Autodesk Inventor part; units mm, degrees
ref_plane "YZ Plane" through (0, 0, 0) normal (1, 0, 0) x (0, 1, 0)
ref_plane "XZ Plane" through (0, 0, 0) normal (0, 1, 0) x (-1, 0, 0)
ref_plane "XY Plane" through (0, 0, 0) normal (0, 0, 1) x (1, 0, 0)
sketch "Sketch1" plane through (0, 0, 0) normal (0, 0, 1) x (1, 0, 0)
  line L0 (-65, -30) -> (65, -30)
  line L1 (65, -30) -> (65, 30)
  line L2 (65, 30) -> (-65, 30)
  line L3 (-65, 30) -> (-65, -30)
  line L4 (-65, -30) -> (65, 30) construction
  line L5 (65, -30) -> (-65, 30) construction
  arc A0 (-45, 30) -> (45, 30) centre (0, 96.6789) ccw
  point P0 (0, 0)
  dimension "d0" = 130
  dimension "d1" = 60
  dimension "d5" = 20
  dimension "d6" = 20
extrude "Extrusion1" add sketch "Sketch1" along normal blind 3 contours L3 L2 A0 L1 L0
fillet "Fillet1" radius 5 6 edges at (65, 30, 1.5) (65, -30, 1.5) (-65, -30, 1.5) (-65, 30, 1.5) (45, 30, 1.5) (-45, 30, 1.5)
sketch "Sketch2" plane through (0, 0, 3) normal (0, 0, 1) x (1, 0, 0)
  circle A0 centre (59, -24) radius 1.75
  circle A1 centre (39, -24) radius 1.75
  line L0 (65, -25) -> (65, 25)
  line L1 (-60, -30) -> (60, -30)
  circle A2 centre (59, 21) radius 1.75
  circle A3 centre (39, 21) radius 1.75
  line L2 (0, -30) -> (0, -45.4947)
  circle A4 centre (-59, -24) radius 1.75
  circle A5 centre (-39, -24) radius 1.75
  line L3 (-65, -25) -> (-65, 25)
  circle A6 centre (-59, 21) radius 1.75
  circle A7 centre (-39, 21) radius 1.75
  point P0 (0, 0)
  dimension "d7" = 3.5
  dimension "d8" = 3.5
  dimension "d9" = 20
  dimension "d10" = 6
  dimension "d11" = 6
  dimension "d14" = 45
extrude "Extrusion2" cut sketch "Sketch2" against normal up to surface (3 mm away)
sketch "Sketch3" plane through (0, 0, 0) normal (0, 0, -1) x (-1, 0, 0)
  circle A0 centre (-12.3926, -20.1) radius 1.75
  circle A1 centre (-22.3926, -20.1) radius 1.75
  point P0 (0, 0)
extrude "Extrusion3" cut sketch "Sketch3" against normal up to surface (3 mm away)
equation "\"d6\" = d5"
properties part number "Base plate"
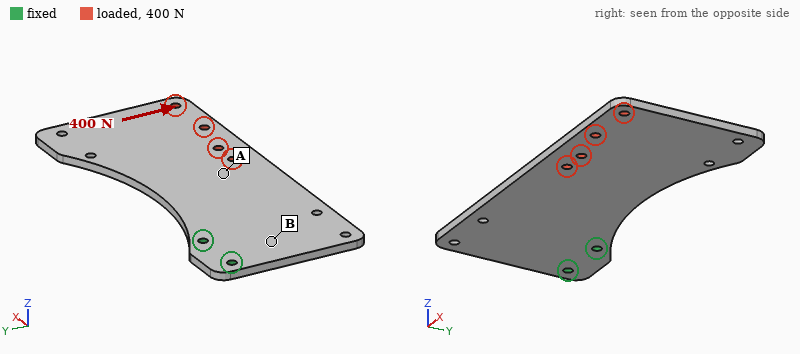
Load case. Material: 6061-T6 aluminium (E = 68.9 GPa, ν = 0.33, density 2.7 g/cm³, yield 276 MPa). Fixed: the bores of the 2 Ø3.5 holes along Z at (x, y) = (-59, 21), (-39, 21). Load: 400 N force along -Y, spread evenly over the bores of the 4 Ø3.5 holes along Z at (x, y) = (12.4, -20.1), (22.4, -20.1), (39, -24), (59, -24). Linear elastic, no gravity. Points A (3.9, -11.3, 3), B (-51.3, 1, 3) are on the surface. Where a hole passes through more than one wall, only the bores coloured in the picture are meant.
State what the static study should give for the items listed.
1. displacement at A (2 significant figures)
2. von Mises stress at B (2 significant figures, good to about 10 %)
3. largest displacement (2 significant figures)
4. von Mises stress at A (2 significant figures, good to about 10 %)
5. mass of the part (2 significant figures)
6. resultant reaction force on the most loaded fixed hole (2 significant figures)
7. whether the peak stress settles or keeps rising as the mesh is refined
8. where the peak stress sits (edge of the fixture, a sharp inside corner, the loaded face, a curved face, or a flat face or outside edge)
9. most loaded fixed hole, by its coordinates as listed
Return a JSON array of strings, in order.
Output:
["0.075 mm", "20 MPa", "0.18 mm", "7.6 MPa", "55 g", "1.7 kN", "keeps rising", "edge of the fixture", "(-39, 21)"]
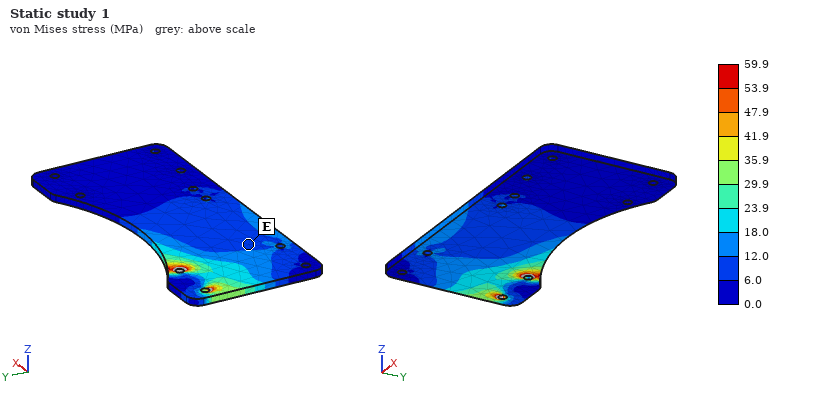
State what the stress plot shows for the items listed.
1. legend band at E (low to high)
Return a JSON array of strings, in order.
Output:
["6.0 to 12.0 MPa"]
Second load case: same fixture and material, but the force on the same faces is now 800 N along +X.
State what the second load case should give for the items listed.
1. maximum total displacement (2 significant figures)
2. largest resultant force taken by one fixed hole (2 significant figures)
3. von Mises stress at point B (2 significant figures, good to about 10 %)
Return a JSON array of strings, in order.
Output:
["0.17 mm", "1.7 kN", "23 MPa"]
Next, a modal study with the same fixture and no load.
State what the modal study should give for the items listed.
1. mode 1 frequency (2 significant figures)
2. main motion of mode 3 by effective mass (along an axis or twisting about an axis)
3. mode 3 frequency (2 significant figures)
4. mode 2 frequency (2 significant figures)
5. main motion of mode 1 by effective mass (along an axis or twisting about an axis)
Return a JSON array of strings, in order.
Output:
["170 Hz", "along Z", "1100 Hz", "540 Hz", "along Z"]
